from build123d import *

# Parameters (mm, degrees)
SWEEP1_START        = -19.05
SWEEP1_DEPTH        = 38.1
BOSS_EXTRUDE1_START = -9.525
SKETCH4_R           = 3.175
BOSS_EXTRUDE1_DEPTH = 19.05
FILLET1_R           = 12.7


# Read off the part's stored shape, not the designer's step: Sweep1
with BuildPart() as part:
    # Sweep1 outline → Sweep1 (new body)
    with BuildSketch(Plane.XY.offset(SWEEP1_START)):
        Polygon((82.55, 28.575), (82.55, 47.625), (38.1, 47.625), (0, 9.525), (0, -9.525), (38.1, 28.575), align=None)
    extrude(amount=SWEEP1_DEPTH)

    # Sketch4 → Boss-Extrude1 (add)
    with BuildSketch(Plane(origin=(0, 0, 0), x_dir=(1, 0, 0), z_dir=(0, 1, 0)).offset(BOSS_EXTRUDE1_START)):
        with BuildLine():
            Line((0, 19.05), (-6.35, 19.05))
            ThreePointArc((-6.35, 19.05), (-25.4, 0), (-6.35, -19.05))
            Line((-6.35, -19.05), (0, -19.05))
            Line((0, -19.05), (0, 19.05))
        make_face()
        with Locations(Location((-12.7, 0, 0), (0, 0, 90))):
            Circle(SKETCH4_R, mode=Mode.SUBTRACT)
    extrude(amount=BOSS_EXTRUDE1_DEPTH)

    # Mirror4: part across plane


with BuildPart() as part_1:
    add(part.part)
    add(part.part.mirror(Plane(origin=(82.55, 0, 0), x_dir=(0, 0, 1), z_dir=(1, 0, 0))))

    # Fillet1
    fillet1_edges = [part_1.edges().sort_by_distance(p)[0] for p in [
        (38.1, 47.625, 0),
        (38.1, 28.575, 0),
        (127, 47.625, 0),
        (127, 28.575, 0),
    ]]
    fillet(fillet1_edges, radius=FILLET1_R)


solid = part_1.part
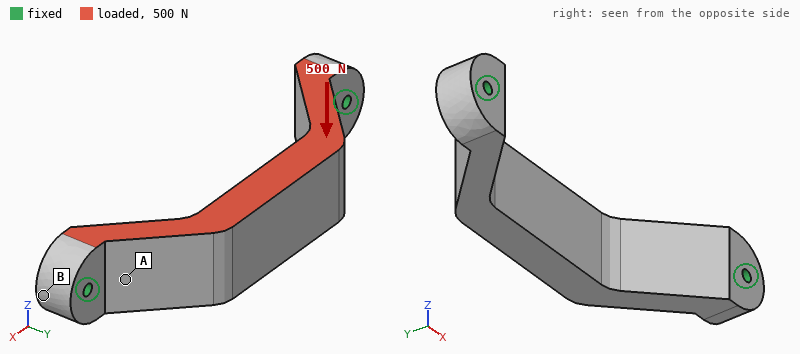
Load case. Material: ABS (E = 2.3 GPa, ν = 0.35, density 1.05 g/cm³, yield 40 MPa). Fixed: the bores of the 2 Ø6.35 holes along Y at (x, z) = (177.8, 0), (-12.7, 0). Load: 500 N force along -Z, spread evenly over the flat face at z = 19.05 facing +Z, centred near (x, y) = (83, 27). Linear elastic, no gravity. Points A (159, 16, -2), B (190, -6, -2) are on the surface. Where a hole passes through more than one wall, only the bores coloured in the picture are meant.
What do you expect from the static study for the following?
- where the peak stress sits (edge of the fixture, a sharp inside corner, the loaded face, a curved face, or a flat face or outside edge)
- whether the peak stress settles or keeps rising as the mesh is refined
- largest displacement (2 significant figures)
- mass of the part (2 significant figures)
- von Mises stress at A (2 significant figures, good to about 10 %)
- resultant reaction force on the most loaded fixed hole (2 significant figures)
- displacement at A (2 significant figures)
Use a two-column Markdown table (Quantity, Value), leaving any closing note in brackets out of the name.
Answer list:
| Quantity | Value |
|---|---|
| where the peak stress sits | edge of the fixture |
| whether the peak stress settles or keeps rising as the mesh is refined | keeps rising |
| largest displacement | 0.44 mm |
| mass of the part | 160 g |
| von Mises stress at A | 2.9 MPa |
| resultant reaction force on the most loaded fixed hole | 250 N |
| displacement at A | 0.13 mm |
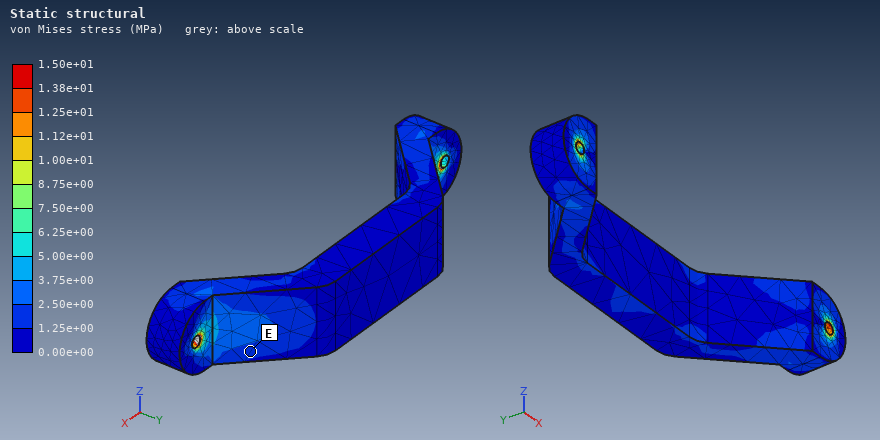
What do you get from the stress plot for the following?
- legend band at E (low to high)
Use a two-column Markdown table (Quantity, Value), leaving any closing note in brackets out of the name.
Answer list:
| Quantity | Value |
|---|---|
| legend band at E | 1.25e+00 to 2.50e+00 MPa |
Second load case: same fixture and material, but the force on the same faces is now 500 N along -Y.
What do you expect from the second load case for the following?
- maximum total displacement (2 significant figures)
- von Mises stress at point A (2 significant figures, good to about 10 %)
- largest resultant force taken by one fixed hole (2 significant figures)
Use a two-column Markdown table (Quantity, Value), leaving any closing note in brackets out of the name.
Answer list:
| Quantity | Value |
|---|---|
| maximum total displacement | 0.26 mm |
| von Mises stress at point A | 1.7 MPa |
| largest resultant force taken by one fixed hole | 330 N |
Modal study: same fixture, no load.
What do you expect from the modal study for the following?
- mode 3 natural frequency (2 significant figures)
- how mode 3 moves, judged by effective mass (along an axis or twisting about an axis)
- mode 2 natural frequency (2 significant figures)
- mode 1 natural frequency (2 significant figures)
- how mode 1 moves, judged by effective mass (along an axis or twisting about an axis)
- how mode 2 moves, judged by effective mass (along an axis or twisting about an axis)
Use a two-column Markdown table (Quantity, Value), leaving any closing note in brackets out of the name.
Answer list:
| Quantity | Value |
|---|---|
| mode 3 natural frequency | 1400 Hz |
| how mode 3 moves, judged by effective mass | along Y |
| mode 2 natural frequency | 1100 Hz |
| mode 1 natural frequency | 530 Hz |
| how mode 1 moves, judged by effective mass | along Z |
| how mode 2 moves, judged by effective mass | along X |
